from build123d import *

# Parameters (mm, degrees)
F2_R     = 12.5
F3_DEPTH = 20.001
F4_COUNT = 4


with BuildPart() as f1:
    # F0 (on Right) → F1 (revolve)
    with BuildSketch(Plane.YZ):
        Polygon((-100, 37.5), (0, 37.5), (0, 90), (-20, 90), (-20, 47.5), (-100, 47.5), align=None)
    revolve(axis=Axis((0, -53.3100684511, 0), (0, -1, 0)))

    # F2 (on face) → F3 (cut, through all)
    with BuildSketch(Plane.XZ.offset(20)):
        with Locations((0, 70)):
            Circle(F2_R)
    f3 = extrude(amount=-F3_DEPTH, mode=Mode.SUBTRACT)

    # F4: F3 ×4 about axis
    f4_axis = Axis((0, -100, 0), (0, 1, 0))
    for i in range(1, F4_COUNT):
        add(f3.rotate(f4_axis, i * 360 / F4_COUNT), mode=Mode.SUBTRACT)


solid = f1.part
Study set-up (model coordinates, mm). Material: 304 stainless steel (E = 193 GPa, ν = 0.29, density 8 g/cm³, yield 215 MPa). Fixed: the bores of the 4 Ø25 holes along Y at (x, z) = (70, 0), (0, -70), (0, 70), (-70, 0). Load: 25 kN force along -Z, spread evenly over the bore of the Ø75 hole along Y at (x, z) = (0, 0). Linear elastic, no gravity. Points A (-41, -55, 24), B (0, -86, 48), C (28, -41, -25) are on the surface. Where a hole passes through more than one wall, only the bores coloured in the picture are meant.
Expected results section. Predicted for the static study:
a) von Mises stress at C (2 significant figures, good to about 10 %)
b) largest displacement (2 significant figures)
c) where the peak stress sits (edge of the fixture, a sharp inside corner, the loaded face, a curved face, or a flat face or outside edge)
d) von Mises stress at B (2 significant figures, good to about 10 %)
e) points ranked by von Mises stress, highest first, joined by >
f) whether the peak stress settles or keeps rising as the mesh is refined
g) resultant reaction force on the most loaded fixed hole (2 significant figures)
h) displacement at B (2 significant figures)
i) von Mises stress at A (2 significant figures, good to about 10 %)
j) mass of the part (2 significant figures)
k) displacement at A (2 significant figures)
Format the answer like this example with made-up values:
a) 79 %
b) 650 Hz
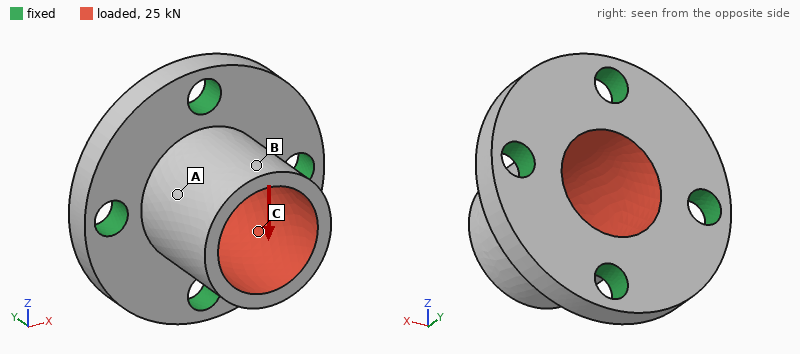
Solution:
a) 18 MPa
b) 20 µm
c) edge of the fixture
d) 4.2 MPa
e) C > A > B
f) keeps rising
g) 11 kN
h) 18 µm
i) 11 MPa
j) 4.8 kg
k) 11 µm
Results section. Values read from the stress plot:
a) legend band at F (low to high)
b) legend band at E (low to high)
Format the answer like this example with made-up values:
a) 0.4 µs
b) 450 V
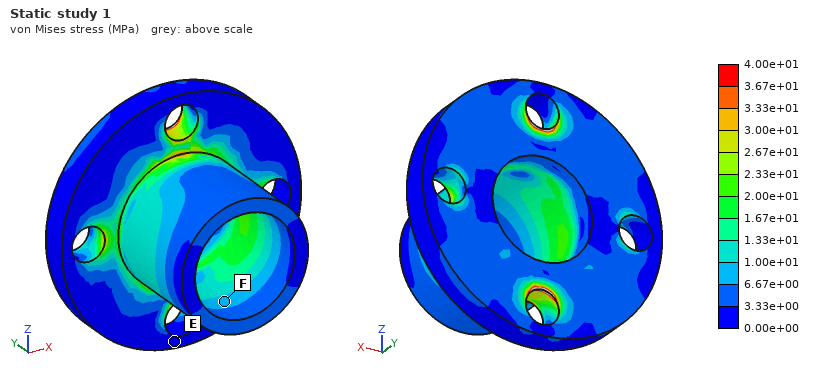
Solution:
a) 6.67e+00 to 1.00e+01 MPa
b) 0.00e+00 to 3.33e+00 MPa
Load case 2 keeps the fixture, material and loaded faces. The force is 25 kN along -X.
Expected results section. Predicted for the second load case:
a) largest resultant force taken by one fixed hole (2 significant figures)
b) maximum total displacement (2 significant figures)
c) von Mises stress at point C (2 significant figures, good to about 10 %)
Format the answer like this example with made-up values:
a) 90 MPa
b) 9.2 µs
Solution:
a) 11 kN
b) 20 µm
c) 17 MPa
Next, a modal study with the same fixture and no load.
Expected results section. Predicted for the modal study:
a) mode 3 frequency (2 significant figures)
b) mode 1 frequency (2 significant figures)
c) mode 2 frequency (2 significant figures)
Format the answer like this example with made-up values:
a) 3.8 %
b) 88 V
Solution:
a) 4400 Hz
b) 4400 Hz
c) 4400 Hz
